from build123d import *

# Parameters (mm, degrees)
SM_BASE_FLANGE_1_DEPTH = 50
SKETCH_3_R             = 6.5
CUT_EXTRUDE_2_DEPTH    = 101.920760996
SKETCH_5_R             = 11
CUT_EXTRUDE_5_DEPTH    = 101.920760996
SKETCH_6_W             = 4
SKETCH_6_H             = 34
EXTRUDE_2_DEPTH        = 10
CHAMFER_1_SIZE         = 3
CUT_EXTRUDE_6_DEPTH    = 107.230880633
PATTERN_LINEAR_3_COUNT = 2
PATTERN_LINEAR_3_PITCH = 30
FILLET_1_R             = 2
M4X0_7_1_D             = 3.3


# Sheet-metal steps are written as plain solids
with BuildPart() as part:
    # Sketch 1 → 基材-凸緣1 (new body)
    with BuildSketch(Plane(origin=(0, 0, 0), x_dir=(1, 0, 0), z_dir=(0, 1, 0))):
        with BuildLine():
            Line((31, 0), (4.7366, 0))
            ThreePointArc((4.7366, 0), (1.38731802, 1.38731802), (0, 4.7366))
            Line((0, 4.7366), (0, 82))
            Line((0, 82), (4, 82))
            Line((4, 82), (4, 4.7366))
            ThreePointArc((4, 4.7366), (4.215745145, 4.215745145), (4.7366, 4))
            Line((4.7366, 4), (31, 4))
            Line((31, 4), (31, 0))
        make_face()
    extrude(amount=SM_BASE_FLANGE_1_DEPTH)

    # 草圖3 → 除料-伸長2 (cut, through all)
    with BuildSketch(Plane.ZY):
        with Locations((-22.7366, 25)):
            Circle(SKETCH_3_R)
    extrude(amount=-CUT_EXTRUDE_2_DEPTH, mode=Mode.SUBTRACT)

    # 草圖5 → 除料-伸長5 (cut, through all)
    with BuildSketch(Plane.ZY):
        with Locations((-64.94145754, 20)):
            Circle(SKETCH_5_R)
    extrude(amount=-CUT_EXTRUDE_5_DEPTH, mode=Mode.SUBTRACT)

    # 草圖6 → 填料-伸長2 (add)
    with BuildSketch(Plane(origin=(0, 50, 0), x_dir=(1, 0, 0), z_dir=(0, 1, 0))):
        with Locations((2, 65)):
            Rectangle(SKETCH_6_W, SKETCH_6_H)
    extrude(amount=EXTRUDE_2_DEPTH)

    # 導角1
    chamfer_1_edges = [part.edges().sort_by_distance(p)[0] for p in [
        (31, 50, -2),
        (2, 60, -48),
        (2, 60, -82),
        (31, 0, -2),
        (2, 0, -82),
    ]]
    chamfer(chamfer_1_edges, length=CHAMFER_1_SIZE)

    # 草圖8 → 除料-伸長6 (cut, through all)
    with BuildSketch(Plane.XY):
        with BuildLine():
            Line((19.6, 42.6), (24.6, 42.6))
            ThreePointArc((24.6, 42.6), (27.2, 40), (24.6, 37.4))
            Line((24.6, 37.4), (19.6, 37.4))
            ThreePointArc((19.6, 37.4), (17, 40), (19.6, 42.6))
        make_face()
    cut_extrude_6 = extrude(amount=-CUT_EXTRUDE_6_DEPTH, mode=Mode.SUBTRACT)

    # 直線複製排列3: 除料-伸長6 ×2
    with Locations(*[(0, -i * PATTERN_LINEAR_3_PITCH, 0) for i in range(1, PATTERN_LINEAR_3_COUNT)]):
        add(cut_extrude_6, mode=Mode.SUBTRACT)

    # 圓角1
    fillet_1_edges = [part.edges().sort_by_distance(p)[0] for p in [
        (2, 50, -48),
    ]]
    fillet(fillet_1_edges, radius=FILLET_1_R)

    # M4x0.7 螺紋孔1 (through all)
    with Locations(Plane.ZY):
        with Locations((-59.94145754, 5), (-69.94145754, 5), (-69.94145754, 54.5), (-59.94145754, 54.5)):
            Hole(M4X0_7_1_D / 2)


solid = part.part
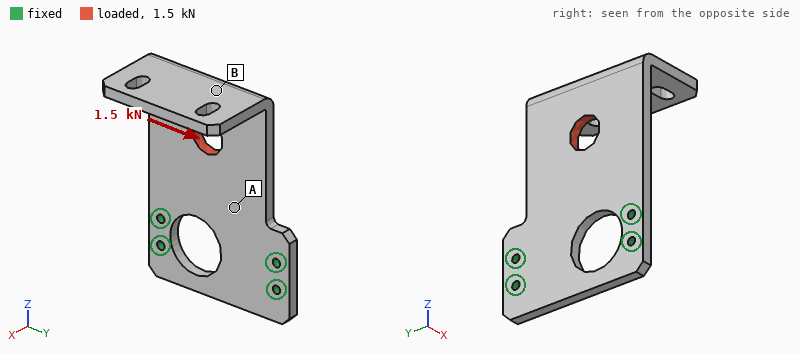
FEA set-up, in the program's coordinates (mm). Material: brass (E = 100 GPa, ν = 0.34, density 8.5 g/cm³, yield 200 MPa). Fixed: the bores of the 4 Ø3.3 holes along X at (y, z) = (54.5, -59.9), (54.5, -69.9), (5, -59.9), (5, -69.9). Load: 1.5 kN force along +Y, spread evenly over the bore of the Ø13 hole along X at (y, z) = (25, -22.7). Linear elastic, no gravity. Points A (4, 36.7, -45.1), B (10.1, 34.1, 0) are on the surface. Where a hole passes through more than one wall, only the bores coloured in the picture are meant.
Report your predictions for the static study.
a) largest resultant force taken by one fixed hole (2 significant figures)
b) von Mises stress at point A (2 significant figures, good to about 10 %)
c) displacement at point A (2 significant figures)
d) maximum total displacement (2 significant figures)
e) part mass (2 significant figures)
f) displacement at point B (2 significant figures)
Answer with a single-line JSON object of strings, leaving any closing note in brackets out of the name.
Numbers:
{"largest resultant force taken by one fixed hole": "1.2 kN", "von Mises stress at point A": "15 MPa", "displacement at point A": "5.0 µm", "maximum total displacement": "23 µm", "part mass": "170 g", "displacement at point B": "22 µm"}
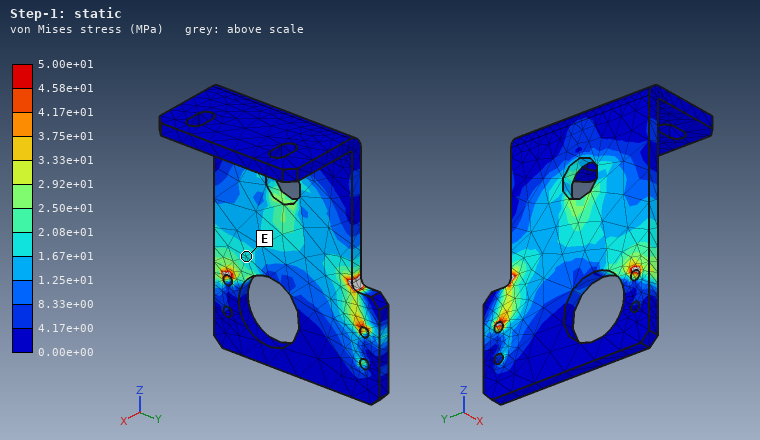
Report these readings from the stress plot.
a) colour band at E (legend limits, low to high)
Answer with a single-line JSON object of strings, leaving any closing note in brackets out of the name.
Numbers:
{"colour band at E": "1.67e+01 to 2.08e+01 MPa"}
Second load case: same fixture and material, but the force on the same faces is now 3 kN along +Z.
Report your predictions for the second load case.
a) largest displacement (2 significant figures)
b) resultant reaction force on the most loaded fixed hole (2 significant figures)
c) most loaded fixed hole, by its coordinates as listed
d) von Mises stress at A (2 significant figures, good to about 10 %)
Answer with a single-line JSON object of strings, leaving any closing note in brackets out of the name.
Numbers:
{"largest displacement": "13 µm", "resultant reaction force on the most loaded fixed hole": "1.5 kN", "most loaded fixed hole, by its coordinates as listed": "(5, -59.9)", "von Mises stress at A": "14 MPa"}
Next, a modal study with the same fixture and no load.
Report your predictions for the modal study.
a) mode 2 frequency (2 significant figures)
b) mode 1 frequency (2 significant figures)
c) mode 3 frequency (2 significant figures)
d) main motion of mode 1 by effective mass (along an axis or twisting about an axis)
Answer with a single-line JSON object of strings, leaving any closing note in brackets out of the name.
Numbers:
{"mode 2 frequency": "890 Hz", "mode 1 frequency": "330 Hz", "mode 3 frequency": "1400 Hz", "main motion of mode 1 by effective mass": "along X"}
